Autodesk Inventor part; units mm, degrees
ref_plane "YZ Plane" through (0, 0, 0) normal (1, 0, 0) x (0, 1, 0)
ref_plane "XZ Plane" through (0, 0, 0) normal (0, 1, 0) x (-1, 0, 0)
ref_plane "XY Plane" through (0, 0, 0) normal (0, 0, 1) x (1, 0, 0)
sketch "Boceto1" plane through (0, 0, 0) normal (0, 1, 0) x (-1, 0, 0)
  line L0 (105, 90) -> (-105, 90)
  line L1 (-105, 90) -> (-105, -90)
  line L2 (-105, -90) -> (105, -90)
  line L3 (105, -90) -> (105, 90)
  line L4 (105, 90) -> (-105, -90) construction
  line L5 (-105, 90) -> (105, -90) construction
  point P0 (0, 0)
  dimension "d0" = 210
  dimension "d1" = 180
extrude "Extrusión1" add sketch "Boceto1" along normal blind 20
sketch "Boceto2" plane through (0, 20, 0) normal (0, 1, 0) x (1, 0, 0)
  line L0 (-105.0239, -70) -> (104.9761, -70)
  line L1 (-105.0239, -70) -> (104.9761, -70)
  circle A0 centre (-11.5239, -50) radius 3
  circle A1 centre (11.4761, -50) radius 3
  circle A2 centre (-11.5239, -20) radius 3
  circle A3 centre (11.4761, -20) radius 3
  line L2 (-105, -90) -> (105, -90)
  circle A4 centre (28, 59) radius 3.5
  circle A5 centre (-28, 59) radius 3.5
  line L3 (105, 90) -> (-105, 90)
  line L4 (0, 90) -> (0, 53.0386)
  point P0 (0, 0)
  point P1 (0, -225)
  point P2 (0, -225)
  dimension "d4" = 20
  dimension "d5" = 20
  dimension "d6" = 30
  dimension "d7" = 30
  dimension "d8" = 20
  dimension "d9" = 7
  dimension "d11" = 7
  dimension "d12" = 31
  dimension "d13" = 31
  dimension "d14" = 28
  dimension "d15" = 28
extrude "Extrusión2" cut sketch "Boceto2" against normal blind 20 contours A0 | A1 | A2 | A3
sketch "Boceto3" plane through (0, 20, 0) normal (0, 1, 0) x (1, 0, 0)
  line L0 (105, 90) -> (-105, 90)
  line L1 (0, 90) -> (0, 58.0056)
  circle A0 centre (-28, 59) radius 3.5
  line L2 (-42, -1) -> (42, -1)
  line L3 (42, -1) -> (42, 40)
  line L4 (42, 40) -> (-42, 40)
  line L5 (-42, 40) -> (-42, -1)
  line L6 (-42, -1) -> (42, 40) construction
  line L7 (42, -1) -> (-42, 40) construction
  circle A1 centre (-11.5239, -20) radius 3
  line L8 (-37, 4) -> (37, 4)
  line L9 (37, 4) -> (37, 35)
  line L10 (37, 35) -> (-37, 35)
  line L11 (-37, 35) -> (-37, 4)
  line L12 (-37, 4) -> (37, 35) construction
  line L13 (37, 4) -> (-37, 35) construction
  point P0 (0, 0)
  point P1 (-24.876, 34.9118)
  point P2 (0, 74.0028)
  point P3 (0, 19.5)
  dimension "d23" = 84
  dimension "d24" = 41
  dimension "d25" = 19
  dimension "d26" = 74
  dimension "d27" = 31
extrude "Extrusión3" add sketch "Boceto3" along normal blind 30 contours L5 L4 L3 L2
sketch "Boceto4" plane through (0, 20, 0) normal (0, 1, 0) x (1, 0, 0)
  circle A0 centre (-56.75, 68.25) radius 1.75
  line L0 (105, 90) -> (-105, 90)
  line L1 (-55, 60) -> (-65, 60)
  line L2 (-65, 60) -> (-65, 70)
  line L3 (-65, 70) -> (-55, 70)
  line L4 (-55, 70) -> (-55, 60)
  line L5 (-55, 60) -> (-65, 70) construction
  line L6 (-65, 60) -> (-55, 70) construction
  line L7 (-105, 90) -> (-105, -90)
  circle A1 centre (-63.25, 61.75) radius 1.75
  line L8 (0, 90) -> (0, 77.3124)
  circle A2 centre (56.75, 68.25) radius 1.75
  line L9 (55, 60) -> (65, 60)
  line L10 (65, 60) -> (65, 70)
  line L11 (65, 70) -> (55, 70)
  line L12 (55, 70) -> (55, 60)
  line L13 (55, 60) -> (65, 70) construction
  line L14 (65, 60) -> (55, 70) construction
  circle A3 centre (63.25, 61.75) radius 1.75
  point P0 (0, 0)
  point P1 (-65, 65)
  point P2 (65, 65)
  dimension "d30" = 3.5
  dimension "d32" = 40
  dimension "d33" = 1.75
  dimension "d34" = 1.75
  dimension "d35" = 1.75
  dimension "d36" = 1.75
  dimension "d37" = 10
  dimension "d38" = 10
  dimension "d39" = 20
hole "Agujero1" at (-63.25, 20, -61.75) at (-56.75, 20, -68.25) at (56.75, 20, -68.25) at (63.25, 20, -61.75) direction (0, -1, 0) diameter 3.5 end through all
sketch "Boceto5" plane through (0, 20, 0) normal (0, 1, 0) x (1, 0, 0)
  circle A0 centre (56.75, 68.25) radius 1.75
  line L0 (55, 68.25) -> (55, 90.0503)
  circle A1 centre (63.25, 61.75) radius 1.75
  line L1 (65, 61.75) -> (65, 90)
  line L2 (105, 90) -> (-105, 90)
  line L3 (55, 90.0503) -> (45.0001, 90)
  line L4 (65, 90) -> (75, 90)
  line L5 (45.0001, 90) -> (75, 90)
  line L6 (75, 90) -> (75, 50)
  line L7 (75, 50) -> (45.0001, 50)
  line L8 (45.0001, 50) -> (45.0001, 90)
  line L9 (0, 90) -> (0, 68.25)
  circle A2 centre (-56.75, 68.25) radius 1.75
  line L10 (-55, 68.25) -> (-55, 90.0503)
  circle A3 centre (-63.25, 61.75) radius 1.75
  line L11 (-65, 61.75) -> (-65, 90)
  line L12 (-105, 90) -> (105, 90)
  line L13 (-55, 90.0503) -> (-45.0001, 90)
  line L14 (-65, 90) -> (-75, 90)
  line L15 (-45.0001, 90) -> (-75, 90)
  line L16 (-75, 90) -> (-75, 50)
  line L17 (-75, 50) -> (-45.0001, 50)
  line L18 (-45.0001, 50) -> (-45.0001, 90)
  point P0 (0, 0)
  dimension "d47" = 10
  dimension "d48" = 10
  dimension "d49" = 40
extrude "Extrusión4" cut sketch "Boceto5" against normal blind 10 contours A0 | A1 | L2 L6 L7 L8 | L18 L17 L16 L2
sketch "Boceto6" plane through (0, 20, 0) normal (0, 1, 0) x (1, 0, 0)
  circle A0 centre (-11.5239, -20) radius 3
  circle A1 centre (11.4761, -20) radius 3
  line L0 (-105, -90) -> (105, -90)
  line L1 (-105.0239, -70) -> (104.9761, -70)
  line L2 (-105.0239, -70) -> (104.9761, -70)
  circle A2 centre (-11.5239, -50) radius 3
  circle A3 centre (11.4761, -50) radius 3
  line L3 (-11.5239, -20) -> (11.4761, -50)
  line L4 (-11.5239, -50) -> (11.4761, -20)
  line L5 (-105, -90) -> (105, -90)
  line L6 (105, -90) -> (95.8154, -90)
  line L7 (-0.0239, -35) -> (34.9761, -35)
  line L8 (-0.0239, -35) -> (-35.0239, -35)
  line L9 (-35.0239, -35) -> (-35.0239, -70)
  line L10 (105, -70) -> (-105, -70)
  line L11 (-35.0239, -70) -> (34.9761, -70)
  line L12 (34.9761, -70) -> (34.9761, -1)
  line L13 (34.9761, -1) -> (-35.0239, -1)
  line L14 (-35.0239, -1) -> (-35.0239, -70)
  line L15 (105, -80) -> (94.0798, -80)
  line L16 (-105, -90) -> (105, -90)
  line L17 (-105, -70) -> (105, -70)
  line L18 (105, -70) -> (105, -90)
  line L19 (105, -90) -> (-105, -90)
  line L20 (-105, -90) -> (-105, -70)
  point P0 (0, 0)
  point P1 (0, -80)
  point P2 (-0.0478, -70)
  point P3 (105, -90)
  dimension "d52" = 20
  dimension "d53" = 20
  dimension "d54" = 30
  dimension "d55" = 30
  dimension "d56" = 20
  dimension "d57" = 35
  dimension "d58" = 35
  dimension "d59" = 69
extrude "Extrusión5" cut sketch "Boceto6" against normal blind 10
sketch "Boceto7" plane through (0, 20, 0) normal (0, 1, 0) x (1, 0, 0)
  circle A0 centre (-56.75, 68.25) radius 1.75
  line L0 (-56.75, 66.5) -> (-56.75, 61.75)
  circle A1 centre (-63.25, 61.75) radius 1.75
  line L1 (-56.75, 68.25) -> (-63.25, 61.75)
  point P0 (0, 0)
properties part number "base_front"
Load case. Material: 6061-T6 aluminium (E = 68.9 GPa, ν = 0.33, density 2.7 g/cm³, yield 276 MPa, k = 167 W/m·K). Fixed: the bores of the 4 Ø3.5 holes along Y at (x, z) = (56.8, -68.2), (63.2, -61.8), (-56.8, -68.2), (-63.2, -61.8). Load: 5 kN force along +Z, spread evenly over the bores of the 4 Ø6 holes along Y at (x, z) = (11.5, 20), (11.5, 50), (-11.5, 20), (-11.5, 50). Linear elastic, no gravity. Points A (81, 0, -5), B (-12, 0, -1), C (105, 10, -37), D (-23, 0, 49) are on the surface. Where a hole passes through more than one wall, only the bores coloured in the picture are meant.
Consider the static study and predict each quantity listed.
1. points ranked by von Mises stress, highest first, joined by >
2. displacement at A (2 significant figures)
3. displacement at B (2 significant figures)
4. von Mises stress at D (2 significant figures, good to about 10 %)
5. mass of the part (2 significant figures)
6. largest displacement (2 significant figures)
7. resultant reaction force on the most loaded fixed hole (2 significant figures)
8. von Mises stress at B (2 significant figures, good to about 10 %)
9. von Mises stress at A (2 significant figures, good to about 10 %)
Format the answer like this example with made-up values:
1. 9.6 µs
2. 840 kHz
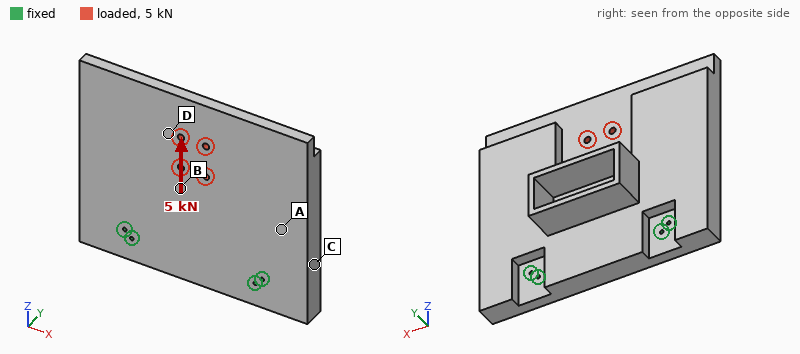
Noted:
1. B > D > A > C
2. 3.8 µm
3. 7.8 µm
4. 3.3 MPa
5. 1.8 kg
6. 23 µm
7. 1.3 kN
8. 5.2 MPa
9. 2.0 MPa
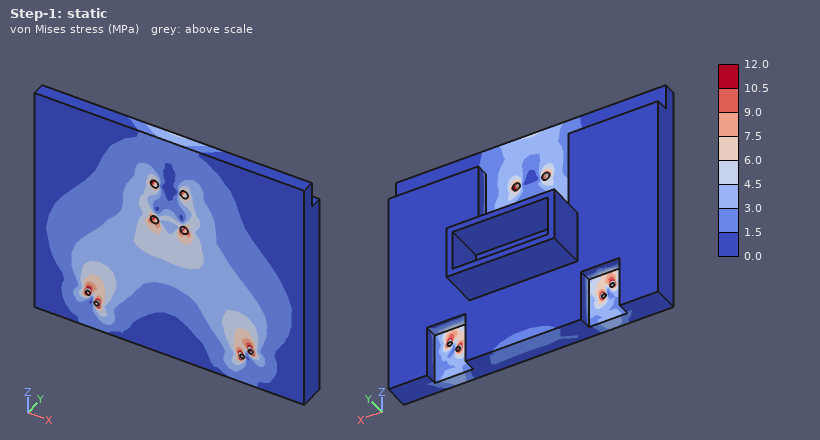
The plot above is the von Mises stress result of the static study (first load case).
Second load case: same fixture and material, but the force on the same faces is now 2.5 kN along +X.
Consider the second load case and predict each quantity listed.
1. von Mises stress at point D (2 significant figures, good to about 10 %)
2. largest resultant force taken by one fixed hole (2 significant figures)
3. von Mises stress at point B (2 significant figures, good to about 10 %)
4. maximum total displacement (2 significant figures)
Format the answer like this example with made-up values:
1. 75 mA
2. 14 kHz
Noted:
1. 2.4 MPa
2. 1.6 kN
3. 3.3 MPa
4. 19 µm
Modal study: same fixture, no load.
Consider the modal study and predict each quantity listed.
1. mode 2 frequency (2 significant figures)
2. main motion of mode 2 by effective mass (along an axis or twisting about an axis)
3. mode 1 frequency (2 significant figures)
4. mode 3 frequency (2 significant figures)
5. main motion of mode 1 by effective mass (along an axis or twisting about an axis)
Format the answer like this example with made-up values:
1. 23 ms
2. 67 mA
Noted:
1. 920 Hz
2. twisting about Z
3. 380 Hz
4. 2300 Hz
5. along Y
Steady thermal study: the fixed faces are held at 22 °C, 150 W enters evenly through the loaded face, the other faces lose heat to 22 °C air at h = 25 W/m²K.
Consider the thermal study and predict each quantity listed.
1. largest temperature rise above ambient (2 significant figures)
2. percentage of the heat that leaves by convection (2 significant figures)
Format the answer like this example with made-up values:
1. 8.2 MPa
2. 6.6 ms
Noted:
1. 42 K
2. 31 %
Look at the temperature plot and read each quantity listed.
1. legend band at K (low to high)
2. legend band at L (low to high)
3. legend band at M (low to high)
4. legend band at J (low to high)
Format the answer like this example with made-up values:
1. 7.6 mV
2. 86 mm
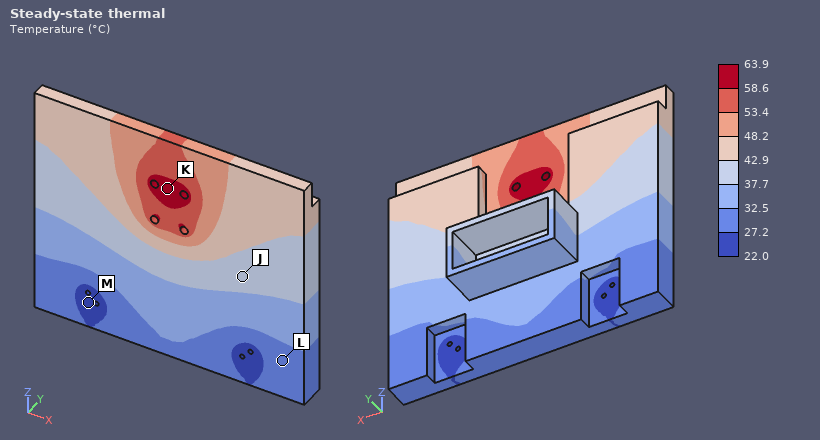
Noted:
1. 58.6 to 63.9 °C
2. 27.2 to 32.5 °C
3. 22.0 to 27.2 °C
4. 37.7 to 42.9 °C
